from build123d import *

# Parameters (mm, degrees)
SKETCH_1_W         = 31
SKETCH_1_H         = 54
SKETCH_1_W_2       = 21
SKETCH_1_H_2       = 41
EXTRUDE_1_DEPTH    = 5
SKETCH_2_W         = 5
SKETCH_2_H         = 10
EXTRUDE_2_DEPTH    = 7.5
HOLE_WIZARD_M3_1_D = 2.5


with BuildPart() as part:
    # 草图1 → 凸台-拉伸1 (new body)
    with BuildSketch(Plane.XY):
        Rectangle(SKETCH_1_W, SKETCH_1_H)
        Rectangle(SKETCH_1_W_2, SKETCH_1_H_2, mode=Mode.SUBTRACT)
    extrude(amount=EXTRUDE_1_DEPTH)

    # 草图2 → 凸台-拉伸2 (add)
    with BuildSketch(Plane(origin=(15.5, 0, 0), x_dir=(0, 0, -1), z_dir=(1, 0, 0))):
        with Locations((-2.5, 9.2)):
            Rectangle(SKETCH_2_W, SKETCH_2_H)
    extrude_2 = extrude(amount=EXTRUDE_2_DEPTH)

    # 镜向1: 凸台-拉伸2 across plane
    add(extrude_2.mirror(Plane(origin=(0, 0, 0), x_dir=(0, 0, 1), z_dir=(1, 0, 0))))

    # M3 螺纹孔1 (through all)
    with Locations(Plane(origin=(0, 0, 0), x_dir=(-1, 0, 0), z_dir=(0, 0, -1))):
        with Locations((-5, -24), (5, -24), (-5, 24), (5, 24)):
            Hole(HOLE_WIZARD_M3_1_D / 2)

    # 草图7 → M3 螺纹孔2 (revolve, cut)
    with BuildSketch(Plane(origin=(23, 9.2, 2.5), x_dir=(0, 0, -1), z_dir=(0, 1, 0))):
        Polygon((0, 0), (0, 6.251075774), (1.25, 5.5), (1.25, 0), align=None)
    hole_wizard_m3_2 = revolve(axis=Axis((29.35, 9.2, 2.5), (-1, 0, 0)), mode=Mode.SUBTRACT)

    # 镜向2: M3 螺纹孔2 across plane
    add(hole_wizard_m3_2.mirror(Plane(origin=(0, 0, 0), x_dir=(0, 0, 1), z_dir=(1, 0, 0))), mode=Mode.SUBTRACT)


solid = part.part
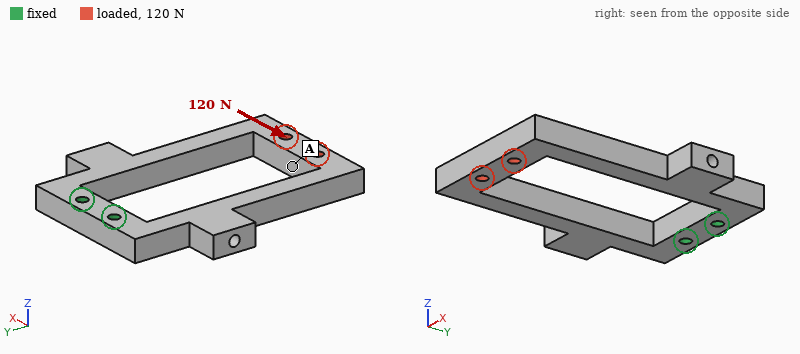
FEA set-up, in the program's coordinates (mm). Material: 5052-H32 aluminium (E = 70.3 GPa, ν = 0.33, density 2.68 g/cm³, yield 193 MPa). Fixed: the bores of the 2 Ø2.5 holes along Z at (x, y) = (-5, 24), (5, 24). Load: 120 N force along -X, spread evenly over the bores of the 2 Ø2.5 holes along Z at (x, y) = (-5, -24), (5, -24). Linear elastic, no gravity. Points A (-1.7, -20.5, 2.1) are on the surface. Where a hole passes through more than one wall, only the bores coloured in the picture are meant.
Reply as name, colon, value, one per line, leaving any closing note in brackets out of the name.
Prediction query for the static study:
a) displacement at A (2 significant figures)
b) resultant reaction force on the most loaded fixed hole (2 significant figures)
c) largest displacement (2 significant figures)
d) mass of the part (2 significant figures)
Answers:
displacement at A: 0.21 mm
resultant reaction force on the most loaded fixed hole: 290 N
largest displacement: 0.22 mm
mass of the part: 12 g
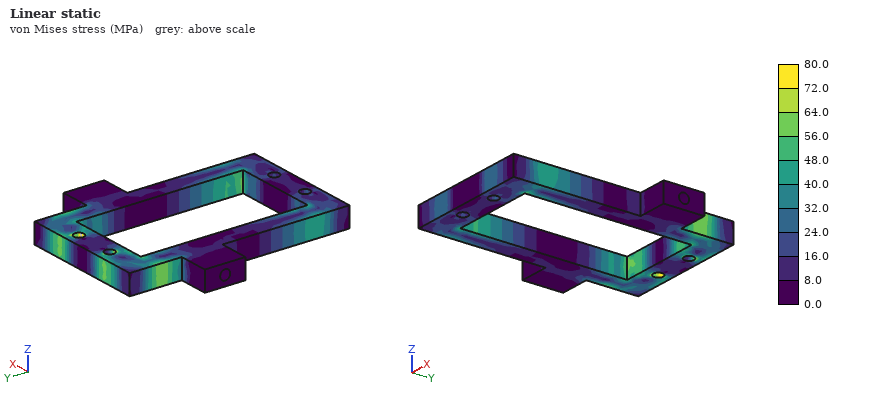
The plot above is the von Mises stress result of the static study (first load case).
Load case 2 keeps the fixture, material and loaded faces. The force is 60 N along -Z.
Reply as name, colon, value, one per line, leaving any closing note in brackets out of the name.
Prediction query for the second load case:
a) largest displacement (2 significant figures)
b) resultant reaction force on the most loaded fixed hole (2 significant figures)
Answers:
largest displacement: 0.41 mm
resultant reaction force on the most loaded fixed hole: 30 N
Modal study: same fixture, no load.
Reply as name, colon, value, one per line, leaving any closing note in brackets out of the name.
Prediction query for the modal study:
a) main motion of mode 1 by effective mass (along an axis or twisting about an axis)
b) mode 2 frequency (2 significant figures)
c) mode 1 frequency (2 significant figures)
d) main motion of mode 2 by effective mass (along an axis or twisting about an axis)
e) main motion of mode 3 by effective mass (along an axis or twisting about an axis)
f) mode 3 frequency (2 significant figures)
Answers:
main motion of mode 1 by effective mass: along Z
mode 2 frequency: 1700 Hz
mode 1 frequency: 1000 Hz
main motion of mode 2 by effective mass: along X
main motion of mode 3 by effective mass: twisting about Y
mode 3 frequency: 2700 Hz
